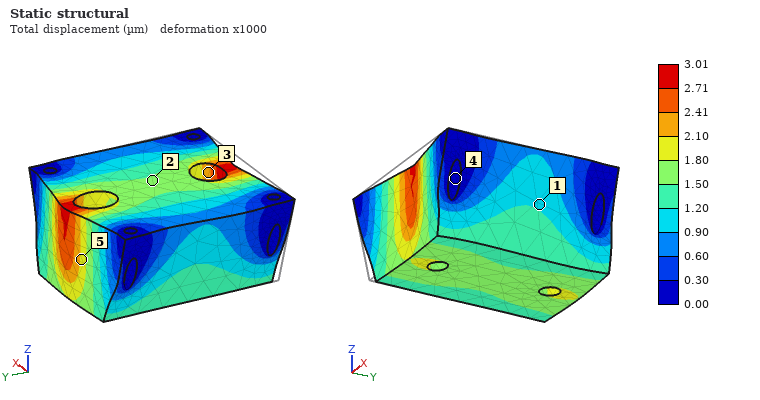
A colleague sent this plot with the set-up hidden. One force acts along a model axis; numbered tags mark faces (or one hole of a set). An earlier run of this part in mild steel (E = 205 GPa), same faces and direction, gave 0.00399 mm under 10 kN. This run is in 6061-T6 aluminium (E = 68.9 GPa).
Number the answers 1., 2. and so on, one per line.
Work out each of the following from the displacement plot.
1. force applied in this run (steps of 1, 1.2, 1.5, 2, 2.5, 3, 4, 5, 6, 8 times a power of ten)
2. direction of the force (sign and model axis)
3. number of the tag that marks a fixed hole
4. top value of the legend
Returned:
1. 2.5 kN
2. +Y
3. 4
4. 3.01 µm
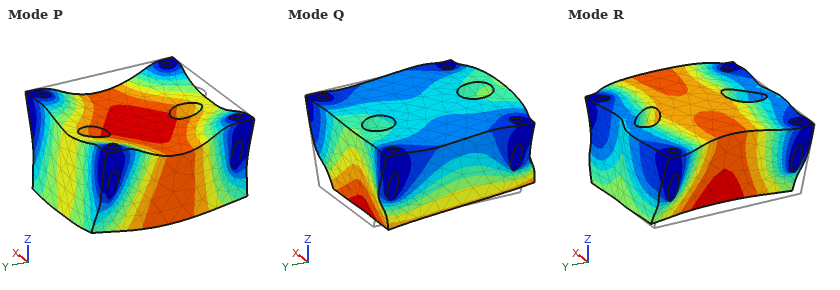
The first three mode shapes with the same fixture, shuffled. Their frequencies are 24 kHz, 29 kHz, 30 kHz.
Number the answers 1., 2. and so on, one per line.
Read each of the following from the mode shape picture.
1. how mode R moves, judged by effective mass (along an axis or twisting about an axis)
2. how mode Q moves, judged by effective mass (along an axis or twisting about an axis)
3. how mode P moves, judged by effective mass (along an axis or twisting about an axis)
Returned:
1. along X
2. along Y
3. along Z
